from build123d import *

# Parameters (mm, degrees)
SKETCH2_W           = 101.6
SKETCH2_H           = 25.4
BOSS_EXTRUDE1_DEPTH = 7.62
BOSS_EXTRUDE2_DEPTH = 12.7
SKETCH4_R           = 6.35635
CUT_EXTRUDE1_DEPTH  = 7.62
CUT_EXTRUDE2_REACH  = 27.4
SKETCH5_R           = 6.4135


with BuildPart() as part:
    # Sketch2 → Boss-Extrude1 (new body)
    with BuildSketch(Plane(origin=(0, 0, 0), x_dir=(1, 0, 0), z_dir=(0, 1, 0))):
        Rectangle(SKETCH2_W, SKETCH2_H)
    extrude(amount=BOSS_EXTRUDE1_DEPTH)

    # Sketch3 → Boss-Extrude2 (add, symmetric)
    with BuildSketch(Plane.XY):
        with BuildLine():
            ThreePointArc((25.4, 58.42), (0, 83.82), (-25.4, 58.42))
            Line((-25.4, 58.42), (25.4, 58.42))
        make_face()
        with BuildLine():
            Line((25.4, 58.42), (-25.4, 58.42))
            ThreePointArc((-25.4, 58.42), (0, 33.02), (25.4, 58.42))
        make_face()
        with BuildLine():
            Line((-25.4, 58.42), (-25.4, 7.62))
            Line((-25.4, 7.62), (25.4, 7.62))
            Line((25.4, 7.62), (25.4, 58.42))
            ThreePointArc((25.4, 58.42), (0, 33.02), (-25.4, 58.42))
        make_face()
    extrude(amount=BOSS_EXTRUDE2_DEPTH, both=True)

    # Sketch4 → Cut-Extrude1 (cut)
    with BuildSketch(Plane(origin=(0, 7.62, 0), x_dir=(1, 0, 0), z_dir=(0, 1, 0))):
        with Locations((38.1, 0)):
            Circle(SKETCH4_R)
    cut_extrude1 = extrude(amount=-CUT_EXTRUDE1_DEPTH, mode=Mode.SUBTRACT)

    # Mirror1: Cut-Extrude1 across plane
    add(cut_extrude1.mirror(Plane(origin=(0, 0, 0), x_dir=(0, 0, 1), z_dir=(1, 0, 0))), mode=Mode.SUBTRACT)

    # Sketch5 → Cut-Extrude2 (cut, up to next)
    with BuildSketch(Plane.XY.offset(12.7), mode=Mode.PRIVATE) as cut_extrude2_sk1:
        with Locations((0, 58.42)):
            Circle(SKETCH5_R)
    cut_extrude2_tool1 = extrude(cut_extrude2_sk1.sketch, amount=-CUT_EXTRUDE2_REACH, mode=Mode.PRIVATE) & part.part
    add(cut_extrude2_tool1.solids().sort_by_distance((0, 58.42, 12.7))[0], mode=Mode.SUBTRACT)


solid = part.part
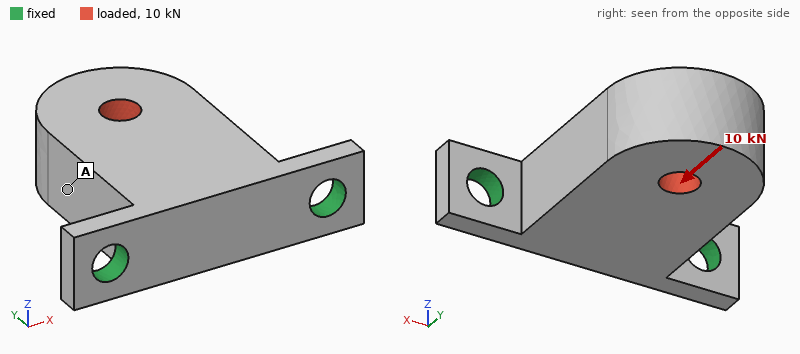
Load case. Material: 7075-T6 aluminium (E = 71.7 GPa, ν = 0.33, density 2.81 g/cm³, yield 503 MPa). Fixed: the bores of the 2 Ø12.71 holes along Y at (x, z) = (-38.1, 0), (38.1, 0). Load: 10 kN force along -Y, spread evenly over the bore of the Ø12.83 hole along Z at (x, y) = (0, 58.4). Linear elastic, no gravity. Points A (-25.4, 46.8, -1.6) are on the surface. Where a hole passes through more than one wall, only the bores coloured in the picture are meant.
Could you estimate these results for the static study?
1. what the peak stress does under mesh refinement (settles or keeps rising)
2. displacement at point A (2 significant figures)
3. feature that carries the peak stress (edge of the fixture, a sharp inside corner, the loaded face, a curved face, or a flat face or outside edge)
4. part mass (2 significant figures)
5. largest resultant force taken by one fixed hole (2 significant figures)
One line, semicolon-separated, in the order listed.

keeps rising; 30 µm; edge of the fixture; 300 g; 5.5 kN
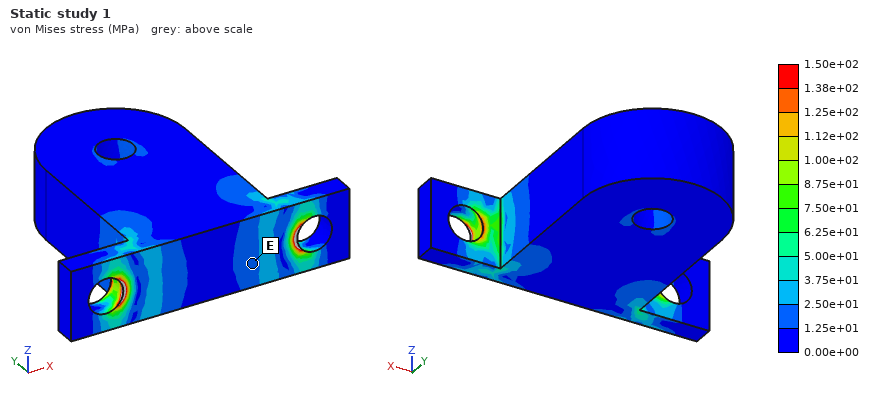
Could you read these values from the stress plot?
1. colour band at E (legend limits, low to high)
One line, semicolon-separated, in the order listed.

1.25e+01 to 2.50e+01 MPa
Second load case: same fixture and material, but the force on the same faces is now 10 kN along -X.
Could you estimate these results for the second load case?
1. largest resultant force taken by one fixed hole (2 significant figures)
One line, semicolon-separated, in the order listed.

11 kN
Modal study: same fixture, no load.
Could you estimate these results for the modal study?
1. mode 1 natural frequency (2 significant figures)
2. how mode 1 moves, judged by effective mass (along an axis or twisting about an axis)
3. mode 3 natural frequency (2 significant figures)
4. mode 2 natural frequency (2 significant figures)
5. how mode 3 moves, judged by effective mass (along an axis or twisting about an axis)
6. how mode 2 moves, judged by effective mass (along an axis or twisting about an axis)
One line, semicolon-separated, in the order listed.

1000 Hz; along Z; 5700 Hz; 3400 Hz; along Y; along X
